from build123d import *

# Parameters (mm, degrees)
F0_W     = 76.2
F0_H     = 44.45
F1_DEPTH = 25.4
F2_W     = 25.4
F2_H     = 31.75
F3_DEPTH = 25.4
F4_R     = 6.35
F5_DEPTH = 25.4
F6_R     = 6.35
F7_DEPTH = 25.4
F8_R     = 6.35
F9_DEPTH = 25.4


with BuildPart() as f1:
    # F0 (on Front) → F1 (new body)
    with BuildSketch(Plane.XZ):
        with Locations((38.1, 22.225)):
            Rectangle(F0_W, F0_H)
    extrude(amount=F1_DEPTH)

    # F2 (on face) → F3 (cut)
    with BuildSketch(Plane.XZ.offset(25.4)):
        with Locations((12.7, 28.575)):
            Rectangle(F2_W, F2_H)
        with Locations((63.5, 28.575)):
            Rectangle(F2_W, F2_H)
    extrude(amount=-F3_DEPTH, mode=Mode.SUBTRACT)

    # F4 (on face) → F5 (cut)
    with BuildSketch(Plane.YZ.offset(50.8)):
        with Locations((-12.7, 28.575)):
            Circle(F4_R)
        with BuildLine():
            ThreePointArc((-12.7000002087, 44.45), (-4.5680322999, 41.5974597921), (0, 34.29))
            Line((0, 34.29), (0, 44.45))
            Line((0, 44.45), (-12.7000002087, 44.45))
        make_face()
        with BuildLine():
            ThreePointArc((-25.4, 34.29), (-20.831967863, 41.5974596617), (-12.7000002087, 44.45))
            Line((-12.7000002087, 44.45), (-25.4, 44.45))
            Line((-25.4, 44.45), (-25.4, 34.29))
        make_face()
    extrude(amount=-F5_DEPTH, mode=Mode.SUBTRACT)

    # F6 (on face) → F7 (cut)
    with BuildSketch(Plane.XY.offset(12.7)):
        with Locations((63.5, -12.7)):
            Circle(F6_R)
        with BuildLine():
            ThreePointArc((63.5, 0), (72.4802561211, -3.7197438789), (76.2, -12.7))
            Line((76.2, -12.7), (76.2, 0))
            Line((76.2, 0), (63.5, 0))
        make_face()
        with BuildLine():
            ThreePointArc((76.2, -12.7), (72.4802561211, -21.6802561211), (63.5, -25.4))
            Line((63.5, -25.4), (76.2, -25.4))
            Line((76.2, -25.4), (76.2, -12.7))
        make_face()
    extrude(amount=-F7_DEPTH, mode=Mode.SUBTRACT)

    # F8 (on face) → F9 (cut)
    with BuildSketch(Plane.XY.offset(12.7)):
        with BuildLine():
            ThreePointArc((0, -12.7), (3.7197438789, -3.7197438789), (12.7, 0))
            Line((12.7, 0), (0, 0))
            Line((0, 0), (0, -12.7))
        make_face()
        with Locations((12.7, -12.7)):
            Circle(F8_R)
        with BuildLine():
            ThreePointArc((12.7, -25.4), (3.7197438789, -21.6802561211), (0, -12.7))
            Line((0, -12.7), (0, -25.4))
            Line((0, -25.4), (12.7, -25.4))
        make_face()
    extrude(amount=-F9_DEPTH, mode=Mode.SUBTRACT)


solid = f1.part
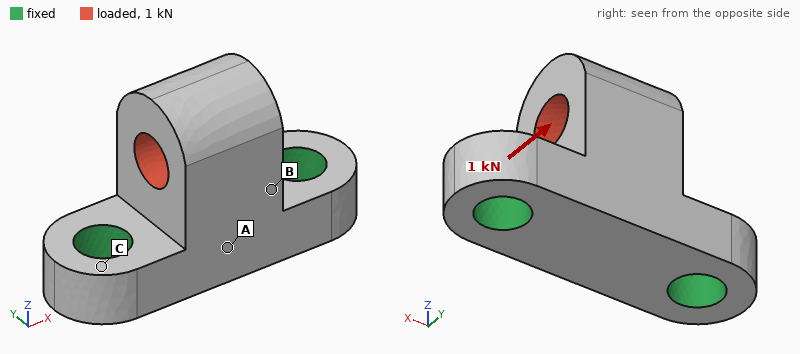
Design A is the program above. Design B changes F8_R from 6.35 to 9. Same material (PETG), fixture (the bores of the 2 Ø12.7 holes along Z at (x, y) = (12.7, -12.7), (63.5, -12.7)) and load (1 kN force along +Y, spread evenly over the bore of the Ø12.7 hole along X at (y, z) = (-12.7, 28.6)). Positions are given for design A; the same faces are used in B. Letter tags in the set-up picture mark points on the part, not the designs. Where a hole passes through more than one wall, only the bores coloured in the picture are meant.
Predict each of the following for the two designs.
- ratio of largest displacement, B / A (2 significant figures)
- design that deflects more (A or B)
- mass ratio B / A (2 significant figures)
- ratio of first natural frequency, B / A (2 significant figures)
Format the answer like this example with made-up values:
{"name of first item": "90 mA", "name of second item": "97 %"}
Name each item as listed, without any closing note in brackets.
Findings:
{"ratio of largest displacement, B / A": "0.87", "design that deflects more": "A", "mass ratio B / A": "0.95", "ratio of first natural frequency, B / A": "1.1"}
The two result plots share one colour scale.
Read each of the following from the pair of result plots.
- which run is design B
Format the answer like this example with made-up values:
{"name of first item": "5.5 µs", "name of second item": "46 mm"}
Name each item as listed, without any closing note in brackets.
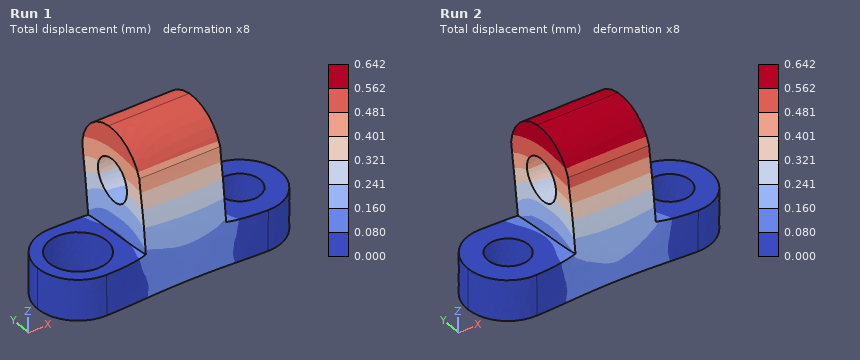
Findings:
{"which run is design B": "Run 1"}
